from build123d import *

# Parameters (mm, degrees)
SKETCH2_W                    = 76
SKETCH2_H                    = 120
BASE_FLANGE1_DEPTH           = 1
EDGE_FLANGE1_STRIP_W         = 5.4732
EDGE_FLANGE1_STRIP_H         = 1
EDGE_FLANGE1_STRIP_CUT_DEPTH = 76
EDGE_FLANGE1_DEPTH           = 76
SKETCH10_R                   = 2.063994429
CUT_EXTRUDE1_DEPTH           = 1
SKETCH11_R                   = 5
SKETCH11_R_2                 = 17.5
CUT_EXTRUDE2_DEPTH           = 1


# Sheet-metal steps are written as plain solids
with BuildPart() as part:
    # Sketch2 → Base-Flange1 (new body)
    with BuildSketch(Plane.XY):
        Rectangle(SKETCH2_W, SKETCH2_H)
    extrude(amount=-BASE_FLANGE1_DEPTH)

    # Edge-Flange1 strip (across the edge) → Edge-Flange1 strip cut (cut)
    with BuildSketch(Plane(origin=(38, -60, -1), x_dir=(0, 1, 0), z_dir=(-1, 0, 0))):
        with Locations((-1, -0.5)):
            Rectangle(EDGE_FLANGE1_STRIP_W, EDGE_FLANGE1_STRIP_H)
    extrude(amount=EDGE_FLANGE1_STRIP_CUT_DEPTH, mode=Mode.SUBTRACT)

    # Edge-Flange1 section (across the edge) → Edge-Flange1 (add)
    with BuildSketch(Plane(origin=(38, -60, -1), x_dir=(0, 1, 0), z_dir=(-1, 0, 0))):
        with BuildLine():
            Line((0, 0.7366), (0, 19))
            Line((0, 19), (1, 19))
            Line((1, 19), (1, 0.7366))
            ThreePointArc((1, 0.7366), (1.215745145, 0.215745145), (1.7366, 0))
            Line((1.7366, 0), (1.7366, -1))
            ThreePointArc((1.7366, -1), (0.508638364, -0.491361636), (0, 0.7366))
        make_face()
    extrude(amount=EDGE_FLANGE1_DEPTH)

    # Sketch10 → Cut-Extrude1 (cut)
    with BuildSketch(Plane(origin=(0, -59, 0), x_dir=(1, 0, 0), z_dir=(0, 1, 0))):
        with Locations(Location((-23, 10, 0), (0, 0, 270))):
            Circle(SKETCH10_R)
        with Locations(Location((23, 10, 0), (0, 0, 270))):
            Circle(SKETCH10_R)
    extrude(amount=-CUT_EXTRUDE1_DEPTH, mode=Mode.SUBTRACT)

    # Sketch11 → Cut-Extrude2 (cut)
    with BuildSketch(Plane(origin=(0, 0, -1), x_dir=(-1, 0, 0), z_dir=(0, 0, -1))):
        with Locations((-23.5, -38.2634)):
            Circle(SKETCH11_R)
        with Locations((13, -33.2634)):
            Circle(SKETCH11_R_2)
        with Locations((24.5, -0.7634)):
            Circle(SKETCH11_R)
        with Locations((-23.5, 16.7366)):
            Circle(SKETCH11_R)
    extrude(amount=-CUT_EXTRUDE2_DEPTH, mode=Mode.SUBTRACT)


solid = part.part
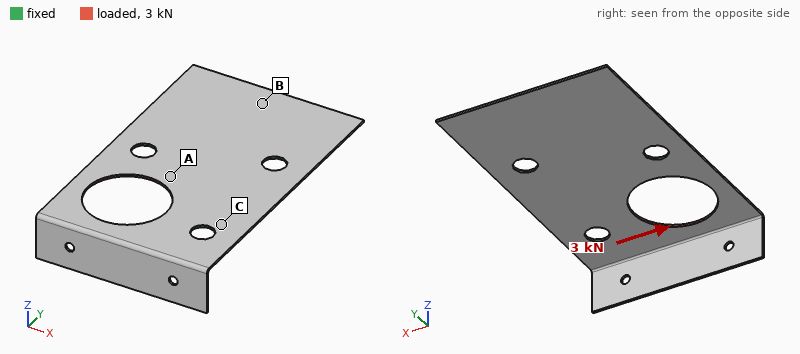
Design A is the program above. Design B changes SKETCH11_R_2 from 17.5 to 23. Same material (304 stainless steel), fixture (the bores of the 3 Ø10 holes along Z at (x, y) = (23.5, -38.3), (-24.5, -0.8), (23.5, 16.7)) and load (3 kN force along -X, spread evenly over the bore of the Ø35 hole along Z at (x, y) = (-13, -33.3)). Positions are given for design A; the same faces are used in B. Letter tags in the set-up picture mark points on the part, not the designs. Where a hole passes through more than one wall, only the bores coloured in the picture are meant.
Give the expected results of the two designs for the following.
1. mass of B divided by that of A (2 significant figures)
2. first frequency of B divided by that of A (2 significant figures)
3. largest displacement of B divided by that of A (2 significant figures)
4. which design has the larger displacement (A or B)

0.92
0.95
4.4
B
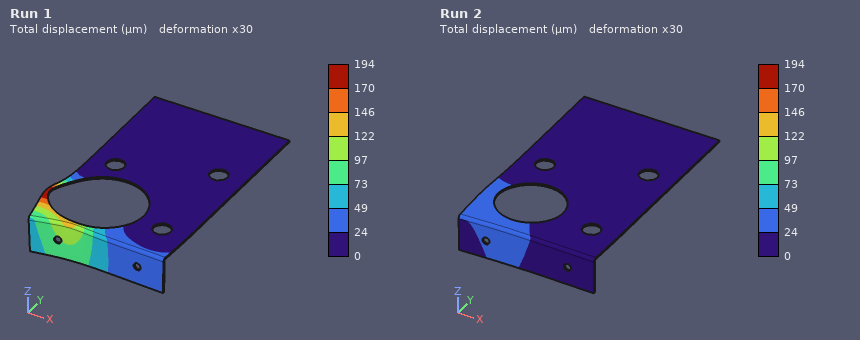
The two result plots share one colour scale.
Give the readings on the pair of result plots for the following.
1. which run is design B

Run 1
